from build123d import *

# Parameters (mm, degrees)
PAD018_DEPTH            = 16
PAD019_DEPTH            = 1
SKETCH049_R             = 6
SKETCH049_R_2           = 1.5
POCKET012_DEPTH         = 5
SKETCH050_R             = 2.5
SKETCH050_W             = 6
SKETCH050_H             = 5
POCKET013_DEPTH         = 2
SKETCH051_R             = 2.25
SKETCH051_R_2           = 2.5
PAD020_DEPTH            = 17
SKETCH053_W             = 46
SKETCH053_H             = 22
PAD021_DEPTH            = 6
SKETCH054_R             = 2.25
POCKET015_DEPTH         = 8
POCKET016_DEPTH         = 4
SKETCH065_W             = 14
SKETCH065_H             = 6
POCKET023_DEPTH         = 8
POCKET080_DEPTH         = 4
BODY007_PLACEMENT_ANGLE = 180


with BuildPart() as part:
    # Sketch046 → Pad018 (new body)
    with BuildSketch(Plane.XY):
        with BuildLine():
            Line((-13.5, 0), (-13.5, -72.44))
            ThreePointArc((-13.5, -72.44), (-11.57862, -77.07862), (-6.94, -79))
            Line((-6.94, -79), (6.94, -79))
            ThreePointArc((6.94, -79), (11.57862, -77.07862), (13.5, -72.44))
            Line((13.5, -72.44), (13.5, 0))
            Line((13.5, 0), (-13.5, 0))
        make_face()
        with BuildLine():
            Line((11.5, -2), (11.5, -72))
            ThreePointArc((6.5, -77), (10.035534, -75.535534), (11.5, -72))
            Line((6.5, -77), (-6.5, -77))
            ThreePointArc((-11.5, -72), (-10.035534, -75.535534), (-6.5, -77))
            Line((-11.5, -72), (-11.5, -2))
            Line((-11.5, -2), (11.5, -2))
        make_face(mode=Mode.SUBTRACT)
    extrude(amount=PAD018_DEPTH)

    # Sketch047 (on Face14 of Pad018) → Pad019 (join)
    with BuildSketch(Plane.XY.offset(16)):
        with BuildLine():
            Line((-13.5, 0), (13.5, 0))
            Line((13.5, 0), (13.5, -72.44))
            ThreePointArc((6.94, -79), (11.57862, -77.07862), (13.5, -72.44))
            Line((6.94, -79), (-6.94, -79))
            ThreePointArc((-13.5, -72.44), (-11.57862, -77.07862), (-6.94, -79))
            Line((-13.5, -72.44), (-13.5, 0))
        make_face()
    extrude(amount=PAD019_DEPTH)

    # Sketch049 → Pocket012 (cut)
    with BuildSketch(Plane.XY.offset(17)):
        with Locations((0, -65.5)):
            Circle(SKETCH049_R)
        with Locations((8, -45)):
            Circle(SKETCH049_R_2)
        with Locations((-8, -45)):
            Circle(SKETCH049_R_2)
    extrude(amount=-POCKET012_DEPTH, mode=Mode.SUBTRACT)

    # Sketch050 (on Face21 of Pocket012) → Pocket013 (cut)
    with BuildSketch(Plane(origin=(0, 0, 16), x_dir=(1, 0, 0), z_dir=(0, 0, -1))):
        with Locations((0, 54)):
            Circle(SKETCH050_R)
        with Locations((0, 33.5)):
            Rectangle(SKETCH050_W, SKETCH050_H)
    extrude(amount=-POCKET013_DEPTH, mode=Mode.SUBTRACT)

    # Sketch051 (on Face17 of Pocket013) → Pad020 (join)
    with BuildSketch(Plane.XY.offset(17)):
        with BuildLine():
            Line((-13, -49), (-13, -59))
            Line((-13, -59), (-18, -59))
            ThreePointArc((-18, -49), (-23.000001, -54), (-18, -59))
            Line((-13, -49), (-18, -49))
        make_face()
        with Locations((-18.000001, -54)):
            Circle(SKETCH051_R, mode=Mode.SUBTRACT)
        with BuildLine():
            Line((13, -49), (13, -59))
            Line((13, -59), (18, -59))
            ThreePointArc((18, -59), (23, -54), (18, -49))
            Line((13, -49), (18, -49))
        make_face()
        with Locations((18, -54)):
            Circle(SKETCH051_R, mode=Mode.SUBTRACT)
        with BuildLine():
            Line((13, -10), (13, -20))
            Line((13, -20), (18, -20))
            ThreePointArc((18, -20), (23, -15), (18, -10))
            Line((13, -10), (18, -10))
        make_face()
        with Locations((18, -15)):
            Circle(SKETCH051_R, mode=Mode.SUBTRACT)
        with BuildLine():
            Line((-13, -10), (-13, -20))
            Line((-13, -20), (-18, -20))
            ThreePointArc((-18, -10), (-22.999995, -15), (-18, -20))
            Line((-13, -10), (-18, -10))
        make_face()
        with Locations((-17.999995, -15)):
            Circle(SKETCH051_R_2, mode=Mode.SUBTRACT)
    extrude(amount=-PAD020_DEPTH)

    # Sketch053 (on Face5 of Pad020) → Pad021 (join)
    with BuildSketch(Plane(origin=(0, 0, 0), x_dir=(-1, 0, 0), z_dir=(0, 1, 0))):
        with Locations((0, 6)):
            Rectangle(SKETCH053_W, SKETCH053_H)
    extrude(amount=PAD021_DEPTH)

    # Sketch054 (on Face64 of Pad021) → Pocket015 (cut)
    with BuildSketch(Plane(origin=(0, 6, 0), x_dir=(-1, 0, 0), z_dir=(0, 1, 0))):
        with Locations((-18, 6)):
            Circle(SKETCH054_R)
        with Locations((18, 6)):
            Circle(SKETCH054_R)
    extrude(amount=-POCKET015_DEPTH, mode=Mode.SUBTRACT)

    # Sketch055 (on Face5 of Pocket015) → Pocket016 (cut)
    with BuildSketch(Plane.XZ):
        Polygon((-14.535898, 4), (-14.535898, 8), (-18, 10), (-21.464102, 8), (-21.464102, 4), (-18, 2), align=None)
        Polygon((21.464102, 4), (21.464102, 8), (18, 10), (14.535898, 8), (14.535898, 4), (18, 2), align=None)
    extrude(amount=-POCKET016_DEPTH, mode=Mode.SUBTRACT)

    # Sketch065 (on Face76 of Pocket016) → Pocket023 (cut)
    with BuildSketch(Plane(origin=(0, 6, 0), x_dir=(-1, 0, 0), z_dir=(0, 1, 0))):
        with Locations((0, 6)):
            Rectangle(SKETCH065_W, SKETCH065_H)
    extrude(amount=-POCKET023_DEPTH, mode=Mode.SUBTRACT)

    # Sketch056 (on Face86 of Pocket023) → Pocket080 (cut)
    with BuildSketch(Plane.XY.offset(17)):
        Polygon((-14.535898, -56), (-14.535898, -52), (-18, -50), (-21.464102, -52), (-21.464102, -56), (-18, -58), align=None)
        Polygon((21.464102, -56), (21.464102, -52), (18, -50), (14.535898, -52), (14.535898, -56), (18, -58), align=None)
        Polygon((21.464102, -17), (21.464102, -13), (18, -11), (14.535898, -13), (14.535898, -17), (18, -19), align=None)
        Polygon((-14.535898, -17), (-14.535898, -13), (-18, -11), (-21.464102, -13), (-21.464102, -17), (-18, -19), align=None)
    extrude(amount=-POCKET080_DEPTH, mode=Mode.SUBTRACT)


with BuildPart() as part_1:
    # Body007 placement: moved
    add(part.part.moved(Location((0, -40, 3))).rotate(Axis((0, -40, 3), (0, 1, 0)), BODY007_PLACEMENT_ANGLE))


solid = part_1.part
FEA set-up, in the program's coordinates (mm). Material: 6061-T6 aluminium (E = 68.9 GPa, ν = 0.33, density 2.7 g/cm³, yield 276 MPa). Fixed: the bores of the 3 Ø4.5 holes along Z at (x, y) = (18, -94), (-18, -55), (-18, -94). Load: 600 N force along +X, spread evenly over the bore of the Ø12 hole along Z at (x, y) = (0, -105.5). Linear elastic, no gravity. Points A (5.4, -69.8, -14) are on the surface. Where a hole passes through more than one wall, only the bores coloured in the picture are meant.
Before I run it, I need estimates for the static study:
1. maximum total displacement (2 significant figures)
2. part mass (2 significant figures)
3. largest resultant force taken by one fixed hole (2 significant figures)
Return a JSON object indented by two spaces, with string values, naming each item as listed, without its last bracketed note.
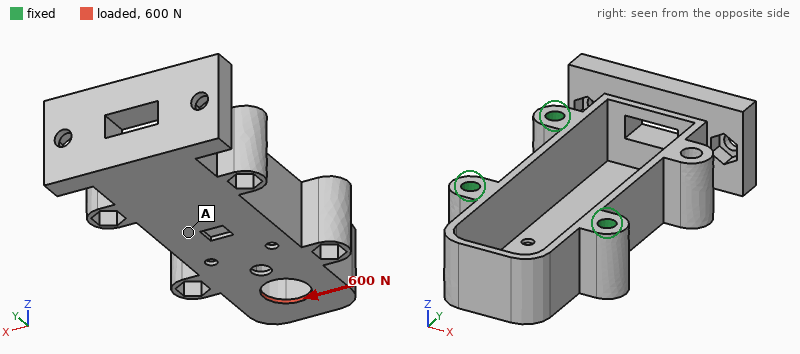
{
  "maximum total displacement": "25 µm",
  "part mass": "47 g",
  "largest resultant force taken by one fixed hole": "360 N"
}
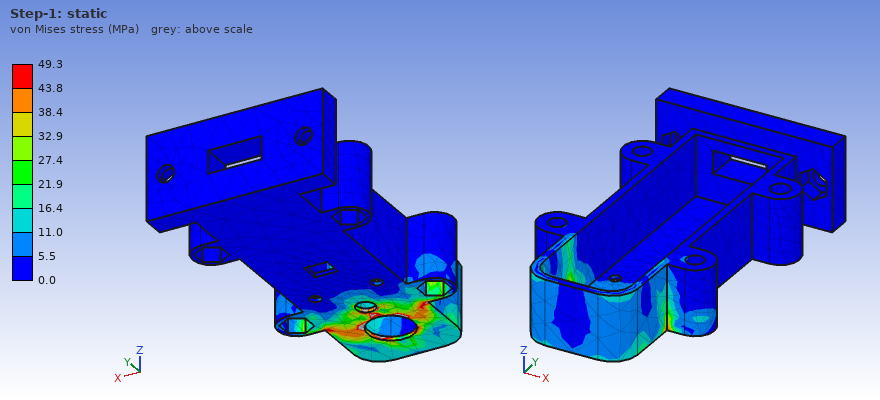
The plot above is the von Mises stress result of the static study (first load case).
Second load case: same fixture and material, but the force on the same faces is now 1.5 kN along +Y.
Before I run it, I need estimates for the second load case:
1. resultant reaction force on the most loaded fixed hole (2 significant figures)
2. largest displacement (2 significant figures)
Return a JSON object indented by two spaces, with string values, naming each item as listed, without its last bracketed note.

{
  "resultant reaction force on the most loaded fixed hole": "680 N",
  "largest displacement": "28 µm"
}
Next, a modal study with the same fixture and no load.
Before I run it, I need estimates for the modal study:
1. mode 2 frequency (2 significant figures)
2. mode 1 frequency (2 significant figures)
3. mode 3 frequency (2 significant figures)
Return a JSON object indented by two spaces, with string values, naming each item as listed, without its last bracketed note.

{
  "mode 2 frequency": "5200 Hz",
  "mode 1 frequency": "2300 Hz",
  "mode 3 frequency": "6100 Hz"
}
